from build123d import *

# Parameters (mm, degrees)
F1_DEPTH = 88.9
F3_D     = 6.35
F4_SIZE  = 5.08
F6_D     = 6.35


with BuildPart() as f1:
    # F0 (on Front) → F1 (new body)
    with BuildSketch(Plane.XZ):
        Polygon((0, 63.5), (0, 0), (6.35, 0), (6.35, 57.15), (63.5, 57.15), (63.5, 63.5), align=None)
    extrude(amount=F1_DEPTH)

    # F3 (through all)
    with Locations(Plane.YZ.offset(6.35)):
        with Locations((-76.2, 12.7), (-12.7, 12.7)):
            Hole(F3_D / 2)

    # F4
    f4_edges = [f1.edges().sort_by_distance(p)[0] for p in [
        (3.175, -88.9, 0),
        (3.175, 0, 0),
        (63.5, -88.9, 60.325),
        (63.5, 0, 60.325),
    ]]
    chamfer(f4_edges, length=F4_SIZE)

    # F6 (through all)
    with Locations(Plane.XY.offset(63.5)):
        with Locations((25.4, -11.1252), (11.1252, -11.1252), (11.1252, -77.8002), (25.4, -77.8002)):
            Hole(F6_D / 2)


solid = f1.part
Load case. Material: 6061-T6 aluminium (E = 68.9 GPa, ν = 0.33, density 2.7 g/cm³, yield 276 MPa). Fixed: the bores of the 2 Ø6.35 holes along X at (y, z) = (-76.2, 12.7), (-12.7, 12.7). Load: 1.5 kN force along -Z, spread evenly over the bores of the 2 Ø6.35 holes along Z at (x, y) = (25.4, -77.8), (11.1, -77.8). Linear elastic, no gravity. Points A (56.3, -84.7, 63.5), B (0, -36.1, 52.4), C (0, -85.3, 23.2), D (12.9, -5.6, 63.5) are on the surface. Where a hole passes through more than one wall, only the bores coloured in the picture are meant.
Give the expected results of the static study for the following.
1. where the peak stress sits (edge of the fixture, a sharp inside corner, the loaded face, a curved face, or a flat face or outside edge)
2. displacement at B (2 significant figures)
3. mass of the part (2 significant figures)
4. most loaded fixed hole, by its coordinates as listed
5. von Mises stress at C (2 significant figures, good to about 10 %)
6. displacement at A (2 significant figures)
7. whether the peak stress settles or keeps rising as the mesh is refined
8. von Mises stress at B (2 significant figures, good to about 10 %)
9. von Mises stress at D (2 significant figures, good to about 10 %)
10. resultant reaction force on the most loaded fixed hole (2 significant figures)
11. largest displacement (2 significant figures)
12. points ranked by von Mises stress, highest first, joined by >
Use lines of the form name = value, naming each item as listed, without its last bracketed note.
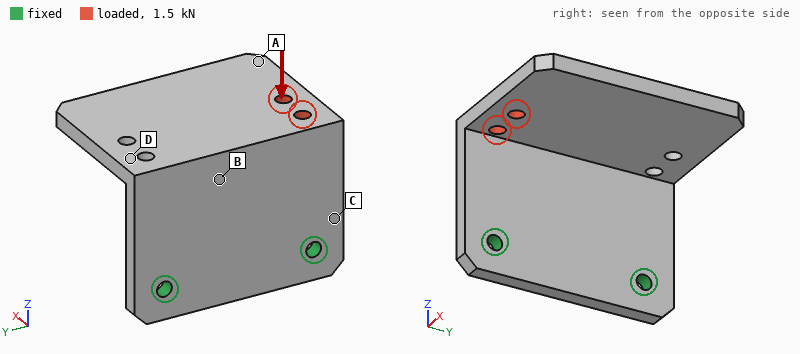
where the peak stress sits = edge of the fixture
displacement at B = 0.15 mm
mass of the part = 180 g
most loaded fixed hole, by its coordinates as listed = (-76.2, 12.7)
von Mises stress at C = 43 MPa
displacement at A = 0.68 mm
whether the peak stress settles or keeps rising as the mesh is refined = keeps rising
von Mises stress at B = 31 MPa
von Mises stress at D = 20 MPa
resultant reaction force on the most loaded fixed hole = 1.5 kN
largest displacement = 0.75 mm
points ranked by von Mises stress, highest first, joined by > = C > B > D > A
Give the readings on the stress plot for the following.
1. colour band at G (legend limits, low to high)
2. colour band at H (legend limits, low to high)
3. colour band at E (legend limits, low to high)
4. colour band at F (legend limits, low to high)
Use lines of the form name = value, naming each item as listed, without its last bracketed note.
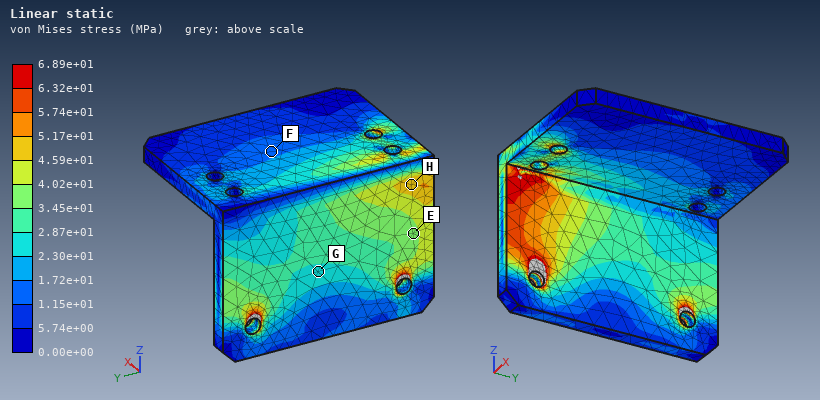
colour band at G = 2.30e+01 to 2.87e+01 MPa
colour band at H = 4.59e+01 to 5.17e+01 MPa
colour band at E = 3.45e+01 to 4.02e+01 MPa
colour band at F = 1.15e+01 to 1.72e+01 MPa
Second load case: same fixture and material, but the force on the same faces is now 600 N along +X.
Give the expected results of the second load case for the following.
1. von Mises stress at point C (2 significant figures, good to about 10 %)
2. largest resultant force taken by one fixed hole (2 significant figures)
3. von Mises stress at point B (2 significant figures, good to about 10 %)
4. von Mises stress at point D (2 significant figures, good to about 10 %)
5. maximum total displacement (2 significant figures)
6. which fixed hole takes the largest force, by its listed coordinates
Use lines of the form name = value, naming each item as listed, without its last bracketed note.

von Mises stress at point C = 64 MPa
largest resultant force taken by one fixed hole = 600 N
von Mises stress at point B = 17 MPa
von Mises stress at point D = 11 MPa
maximum total displacement = 0.50 mm
which fixed hole takes the largest force, by its listed coordinates = (-76.2, 12.7)
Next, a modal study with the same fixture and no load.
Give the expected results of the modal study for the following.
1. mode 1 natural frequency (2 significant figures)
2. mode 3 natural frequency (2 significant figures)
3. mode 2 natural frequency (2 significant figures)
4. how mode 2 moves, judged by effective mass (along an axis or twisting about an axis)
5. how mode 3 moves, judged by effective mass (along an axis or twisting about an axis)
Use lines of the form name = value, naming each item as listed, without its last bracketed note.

mode 1 natural frequency = 580 Hz
mode 3 natural frequency = 1600 Hz
mode 2 natural frequency = 1100 Hz
how mode 2 moves, judged by effective mass = along Y
how mode 3 moves, judged by effective mass = along X
